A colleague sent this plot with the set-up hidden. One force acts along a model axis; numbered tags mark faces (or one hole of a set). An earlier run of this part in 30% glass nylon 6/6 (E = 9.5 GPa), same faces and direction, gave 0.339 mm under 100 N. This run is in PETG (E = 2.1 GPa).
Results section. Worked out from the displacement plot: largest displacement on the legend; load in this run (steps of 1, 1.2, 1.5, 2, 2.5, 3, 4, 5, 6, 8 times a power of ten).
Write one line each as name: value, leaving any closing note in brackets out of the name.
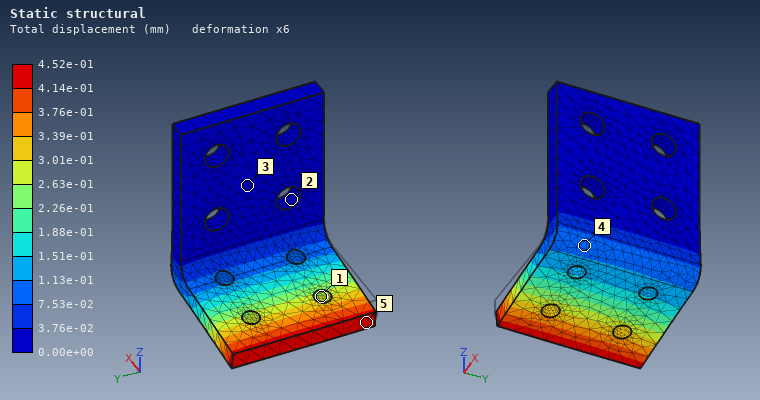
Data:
largest displacement on the legend: 4.52e-01 mm
load in this run: 30 N
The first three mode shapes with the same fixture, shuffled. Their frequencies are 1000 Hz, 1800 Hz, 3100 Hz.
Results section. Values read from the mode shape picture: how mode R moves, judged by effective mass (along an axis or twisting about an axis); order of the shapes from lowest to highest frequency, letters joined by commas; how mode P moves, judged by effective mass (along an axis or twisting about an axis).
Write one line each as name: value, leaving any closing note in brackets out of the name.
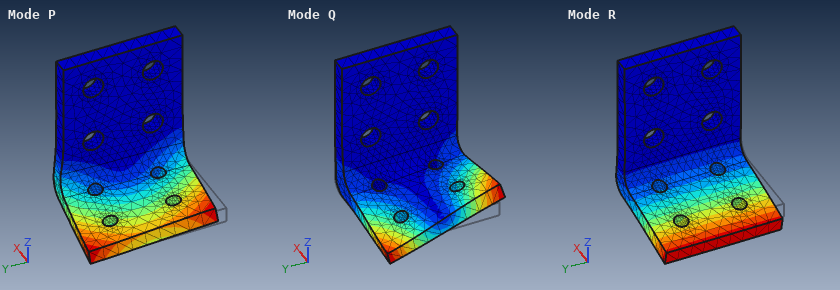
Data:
how mode R moves, judged by effective mass: along Z
order of the shapes from lowest to highest frequency, letters joined by commas: R, P, Q
how mode P moves, judged by effective mass: along Y
